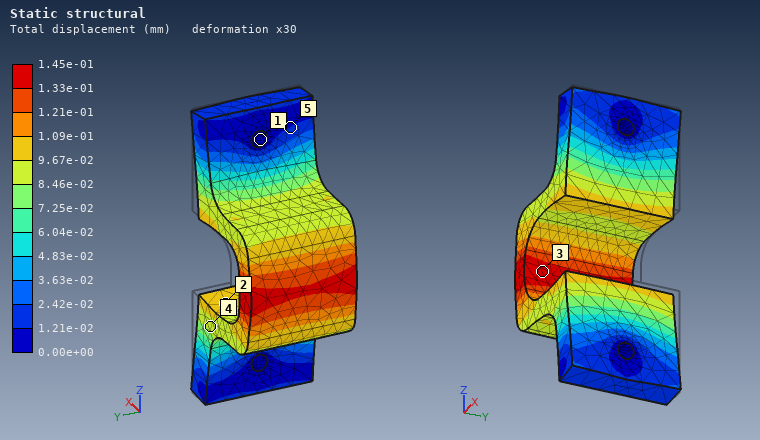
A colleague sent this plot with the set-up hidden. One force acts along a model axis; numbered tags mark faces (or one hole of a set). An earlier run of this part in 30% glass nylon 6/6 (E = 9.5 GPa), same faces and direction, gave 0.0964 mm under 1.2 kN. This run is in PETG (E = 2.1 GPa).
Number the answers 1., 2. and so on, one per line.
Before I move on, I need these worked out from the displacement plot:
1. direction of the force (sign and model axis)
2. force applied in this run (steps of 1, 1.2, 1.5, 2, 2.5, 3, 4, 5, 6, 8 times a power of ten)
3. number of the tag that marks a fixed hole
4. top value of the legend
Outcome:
1. -X
2. 400 N
3. 1
4. 1.45e-01 mm
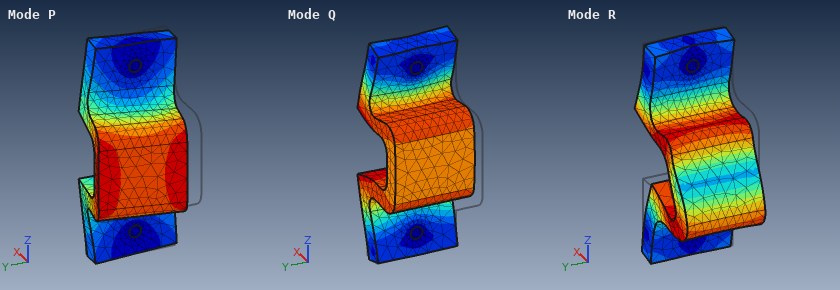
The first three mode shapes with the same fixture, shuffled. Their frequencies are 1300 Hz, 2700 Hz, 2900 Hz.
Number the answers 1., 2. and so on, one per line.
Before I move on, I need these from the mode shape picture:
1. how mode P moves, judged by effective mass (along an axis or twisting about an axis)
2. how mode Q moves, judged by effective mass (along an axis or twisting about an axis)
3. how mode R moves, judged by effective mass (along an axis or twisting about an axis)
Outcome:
1. along Y
2. along X
3. along Z
